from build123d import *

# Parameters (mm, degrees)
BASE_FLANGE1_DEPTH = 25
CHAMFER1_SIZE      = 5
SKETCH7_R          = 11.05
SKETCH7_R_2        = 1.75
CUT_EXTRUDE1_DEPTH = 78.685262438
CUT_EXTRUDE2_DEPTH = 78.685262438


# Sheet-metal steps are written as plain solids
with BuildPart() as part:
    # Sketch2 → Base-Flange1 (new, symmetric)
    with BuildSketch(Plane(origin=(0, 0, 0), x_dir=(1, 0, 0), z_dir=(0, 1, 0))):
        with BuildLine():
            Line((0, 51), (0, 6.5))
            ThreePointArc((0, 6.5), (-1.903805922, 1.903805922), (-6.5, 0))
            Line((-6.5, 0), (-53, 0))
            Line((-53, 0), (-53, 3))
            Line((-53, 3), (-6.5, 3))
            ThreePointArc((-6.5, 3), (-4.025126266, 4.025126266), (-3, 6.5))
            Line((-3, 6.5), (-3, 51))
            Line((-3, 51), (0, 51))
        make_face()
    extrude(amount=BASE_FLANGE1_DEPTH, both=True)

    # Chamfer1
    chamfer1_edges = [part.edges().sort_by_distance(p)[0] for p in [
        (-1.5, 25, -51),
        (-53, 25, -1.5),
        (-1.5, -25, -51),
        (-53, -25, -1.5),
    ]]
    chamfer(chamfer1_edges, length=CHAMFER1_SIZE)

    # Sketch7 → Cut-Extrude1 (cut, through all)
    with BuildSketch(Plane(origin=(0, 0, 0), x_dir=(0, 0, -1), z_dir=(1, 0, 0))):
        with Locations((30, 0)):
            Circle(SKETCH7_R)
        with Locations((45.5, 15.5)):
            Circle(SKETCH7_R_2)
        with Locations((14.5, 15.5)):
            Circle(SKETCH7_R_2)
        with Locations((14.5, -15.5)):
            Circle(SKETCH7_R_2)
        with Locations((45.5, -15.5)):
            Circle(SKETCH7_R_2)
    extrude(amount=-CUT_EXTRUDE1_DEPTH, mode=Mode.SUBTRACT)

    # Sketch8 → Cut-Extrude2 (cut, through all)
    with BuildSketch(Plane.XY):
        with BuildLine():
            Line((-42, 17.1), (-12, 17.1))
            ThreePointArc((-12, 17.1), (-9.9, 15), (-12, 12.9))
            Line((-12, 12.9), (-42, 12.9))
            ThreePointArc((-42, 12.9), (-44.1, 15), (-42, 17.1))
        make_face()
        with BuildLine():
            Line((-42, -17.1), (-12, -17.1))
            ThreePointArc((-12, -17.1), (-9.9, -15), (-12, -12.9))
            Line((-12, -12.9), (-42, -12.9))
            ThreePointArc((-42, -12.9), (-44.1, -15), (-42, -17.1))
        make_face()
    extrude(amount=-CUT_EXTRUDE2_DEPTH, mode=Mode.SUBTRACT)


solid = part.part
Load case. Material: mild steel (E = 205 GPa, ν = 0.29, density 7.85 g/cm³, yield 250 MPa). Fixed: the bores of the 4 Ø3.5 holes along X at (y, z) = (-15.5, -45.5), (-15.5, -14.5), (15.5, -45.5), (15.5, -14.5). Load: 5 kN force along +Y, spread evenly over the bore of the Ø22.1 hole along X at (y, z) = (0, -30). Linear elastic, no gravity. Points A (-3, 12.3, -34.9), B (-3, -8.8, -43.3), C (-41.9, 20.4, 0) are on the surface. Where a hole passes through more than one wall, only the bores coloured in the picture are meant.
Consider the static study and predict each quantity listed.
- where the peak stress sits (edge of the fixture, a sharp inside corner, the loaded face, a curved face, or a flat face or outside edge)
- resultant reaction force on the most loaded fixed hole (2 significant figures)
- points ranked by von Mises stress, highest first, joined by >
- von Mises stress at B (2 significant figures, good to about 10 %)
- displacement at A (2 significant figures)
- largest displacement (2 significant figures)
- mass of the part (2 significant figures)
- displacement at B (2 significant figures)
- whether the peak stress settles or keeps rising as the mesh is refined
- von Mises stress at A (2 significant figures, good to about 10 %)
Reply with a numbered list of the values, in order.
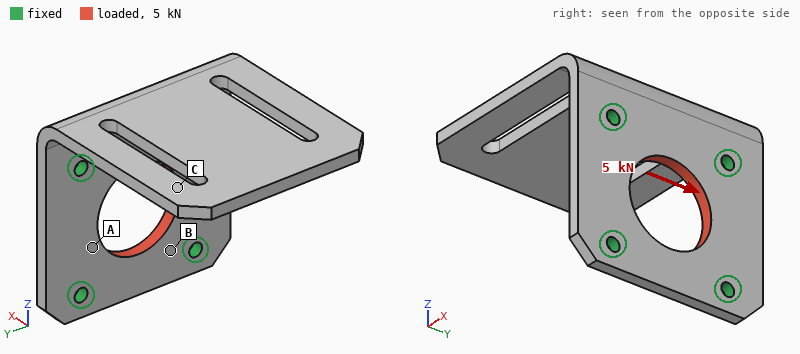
1. edge of the fixture
2. 1.3 kN
3. B > A > C
4. 32 MPa
5. 3.1 µm
6. 3.8 µm
7. 99 g
8. 1.2 µm
9. keeps rising
10. 22 MPa
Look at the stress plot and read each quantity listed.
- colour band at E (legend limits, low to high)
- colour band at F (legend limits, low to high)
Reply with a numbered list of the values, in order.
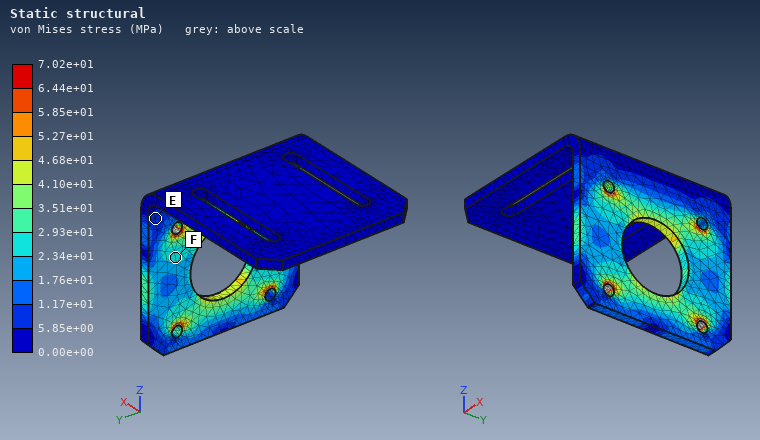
1. 5.85e+00 to 1.17e+01 MPa
2. 2.34e+01 to 2.93e+01 MPa
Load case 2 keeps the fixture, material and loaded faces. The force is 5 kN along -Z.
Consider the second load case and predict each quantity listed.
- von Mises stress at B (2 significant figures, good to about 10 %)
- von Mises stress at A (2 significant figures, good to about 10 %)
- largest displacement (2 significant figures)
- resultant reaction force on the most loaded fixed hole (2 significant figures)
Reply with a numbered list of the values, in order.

1. 34 MPa
2. 39 MPa
3. 5.0 µm
4. 1.3 kN
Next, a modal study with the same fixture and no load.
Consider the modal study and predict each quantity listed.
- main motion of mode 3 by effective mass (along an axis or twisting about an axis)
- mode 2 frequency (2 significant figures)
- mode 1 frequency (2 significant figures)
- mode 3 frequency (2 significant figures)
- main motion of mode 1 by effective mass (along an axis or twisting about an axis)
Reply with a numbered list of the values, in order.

1. along Y
2. 1800 Hz
3. 700 Hz
4. 2700 Hz
5. along Z
